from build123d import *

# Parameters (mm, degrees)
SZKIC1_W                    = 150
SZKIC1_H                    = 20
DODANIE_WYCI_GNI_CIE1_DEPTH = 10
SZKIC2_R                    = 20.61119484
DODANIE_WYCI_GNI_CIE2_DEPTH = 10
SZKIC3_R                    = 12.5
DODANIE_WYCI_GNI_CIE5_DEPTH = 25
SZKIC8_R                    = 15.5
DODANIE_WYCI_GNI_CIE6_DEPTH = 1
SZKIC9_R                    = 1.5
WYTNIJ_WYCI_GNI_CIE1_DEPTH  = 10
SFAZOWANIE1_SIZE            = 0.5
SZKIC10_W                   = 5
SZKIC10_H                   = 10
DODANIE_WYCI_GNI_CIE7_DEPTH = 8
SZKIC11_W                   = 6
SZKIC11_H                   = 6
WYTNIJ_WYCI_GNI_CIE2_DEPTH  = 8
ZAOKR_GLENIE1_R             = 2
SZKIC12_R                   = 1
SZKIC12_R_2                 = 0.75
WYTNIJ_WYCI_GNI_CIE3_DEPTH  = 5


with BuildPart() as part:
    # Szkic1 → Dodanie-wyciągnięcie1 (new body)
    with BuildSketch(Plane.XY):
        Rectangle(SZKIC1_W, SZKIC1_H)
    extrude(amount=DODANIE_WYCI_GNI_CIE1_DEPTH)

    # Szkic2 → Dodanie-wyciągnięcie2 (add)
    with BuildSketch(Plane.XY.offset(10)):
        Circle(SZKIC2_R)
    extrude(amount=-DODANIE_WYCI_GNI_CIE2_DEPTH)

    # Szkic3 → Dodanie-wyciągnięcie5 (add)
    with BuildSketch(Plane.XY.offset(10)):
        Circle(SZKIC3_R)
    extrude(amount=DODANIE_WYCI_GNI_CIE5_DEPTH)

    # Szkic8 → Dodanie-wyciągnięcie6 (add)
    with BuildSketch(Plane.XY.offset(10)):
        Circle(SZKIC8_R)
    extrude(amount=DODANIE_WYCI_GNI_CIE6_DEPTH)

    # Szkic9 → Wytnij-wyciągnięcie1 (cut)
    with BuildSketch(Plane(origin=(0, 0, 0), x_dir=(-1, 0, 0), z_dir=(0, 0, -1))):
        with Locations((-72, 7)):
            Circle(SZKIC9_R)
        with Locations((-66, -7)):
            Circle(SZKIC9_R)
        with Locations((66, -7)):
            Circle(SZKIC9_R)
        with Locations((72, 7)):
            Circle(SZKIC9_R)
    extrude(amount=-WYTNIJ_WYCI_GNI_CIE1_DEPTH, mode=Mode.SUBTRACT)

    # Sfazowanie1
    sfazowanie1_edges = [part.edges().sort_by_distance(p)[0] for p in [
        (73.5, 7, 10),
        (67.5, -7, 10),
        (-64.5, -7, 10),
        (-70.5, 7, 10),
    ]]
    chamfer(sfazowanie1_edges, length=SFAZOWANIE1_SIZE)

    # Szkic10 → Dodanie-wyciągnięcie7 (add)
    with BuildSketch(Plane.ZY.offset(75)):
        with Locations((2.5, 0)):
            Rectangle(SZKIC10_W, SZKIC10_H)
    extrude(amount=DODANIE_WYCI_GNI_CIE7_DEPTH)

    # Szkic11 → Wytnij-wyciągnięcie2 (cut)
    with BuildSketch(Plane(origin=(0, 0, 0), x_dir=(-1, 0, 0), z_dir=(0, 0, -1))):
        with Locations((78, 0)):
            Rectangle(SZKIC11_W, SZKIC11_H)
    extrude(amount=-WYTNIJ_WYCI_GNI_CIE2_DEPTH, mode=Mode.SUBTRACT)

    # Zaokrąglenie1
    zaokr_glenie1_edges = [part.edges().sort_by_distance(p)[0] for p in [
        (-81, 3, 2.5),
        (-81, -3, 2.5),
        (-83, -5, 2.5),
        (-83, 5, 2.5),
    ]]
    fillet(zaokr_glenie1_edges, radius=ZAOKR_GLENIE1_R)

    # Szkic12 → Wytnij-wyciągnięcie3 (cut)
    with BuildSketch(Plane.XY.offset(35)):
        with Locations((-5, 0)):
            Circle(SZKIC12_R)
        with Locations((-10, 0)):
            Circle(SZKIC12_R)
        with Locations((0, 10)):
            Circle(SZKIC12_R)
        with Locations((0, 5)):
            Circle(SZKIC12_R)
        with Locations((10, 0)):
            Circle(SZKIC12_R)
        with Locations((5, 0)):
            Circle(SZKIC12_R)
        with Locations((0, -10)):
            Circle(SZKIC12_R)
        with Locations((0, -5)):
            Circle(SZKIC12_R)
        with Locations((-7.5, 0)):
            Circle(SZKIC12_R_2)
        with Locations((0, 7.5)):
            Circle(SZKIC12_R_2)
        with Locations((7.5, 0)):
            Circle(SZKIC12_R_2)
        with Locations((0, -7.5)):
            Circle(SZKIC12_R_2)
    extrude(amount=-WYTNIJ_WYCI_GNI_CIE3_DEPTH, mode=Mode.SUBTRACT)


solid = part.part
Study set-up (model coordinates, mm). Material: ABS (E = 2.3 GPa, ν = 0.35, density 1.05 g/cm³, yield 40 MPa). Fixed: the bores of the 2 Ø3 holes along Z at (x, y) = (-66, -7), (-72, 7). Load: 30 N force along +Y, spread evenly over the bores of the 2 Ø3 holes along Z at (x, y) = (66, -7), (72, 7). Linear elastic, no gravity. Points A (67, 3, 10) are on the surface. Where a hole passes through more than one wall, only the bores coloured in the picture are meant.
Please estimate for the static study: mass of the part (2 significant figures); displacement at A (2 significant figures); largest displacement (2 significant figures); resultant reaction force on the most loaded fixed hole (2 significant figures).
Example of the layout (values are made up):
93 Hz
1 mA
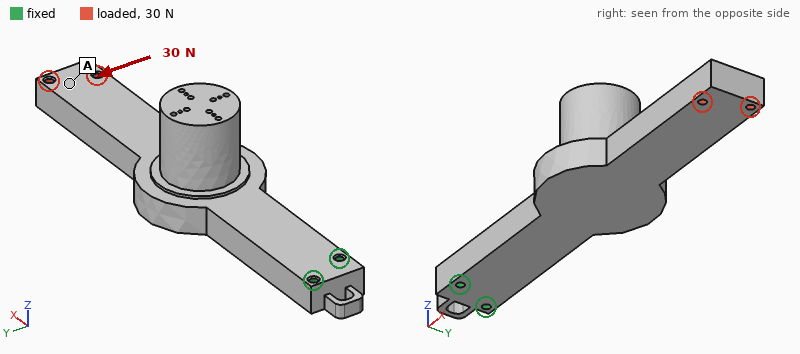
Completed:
50 g
1.5 mm
1.6 mm
270 N
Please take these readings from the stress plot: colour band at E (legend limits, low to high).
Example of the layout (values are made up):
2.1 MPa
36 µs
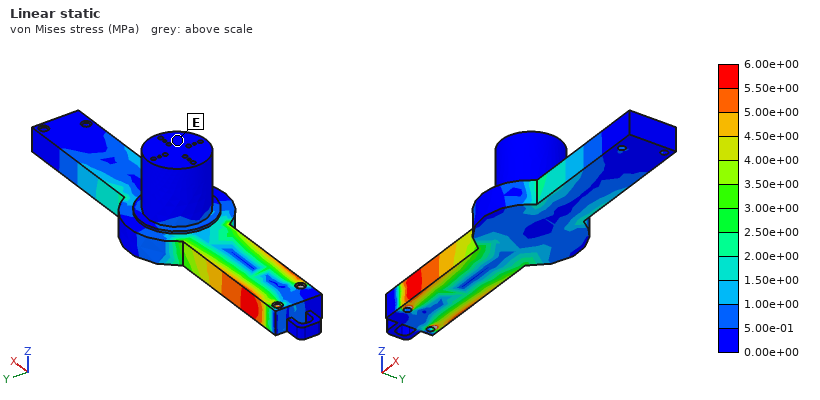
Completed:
0.00e+00 to 5.00e-01 MPa
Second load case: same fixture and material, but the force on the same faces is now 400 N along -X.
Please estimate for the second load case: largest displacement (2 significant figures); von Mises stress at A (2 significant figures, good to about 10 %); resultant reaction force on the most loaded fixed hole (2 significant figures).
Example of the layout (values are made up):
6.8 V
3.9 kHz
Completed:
0.35 mm
1.4 MPa
200 N
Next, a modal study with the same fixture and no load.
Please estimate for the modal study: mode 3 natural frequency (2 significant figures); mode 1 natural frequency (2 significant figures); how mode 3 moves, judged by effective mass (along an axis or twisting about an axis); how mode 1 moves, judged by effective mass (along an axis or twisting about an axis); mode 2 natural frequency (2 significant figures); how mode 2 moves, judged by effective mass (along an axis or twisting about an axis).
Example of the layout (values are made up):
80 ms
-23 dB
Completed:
530 Hz
110 Hz
twisting about X
along Z
210 Hz
along Y
